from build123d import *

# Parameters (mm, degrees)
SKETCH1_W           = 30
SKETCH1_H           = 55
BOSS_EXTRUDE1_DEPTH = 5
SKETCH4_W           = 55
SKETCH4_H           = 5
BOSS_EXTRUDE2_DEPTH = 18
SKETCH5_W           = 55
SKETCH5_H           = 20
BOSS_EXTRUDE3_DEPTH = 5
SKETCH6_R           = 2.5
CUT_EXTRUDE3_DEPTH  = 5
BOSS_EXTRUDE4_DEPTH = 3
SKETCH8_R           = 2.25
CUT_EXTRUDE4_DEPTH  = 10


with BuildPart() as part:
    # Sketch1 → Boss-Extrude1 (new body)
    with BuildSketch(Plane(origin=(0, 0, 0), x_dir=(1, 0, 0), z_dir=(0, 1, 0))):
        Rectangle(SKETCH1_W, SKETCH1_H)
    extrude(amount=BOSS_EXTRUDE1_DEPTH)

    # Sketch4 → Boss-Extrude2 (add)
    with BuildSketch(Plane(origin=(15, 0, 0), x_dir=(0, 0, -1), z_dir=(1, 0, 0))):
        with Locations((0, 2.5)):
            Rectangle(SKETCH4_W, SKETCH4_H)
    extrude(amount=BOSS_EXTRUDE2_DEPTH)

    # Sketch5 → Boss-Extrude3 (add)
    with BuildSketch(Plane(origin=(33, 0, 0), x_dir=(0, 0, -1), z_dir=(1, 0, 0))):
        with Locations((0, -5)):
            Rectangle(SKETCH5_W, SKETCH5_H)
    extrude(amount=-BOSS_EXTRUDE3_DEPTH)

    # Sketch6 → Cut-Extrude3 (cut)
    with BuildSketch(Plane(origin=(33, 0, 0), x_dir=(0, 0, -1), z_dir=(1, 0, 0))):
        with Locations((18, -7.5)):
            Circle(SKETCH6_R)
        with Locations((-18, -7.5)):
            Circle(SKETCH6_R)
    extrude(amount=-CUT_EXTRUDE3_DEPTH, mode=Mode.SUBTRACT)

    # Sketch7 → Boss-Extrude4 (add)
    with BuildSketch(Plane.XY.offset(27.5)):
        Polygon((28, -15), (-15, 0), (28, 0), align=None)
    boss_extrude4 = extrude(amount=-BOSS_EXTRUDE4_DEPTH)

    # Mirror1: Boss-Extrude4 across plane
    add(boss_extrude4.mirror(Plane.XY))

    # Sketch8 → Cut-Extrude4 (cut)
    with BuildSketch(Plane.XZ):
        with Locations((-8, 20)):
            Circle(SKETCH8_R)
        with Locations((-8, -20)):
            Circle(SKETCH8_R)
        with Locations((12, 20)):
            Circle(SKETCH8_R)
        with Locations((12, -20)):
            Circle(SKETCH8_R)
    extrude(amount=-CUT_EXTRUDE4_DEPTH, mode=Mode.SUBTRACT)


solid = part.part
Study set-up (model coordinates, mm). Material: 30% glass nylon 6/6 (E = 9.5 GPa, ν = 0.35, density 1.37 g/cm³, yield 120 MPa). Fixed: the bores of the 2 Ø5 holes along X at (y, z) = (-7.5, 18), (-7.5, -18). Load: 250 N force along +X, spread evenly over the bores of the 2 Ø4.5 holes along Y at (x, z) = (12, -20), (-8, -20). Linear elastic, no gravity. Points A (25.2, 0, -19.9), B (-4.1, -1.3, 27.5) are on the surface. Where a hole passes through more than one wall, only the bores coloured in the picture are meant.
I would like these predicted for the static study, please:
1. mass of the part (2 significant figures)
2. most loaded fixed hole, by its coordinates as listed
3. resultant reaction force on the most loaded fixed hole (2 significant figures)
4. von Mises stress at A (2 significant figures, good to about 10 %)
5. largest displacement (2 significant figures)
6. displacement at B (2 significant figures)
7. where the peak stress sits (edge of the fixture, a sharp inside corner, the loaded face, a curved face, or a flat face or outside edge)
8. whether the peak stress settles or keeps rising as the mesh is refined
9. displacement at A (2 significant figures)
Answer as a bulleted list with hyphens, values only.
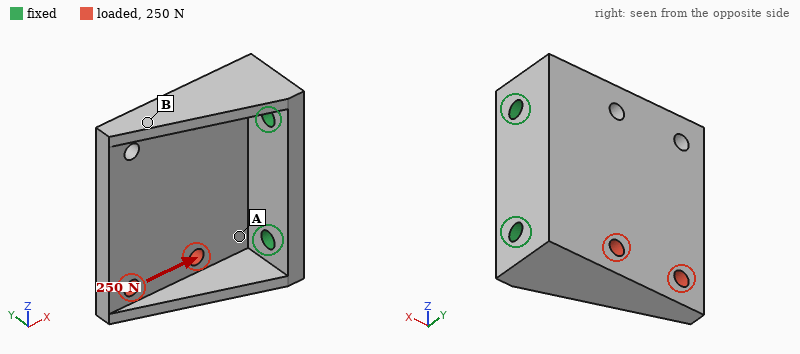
- 26 g
- (-7.5, -18)
- 250 N
- 5.0 MPa
- 0.15 mm
- 0.036 mm
- edge of the fixture
- keeps rising
- 0.029 mm
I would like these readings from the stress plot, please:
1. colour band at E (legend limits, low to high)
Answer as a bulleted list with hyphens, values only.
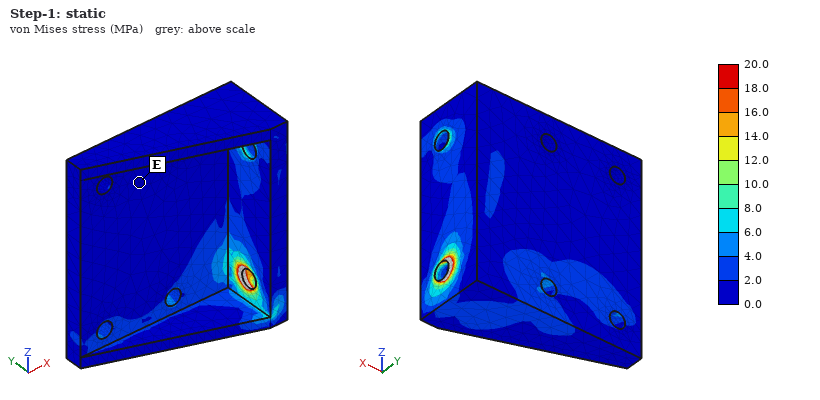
- 0.0 to 2.0 MPa
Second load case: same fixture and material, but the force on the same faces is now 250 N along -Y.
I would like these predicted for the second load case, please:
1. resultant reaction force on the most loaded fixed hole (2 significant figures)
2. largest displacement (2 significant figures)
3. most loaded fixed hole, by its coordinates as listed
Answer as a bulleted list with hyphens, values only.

- 250 N
- 0.61 mm
- (-7.5, -18)
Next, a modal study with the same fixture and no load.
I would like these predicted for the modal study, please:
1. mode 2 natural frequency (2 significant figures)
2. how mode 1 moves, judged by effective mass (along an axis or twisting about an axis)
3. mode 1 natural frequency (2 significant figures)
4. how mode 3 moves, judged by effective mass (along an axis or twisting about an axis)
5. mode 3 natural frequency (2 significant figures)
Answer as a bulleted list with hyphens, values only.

- 2100 Hz
- along Y
- 1200 Hz
- along Z
- 4200 Hz
